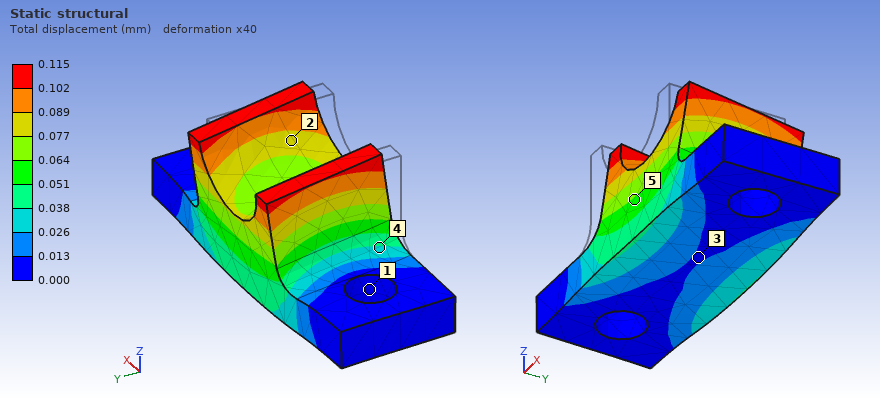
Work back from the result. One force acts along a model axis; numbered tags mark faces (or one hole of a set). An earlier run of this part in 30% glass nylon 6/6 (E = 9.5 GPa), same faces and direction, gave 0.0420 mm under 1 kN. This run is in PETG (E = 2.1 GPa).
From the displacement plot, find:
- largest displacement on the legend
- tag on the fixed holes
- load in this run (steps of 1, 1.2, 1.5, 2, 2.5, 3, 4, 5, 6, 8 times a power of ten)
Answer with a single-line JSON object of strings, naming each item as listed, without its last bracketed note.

{"largest displacement on the legend": "0.115 mm", "tag on the fixed holes": "1", "load in this run": "600 N"}
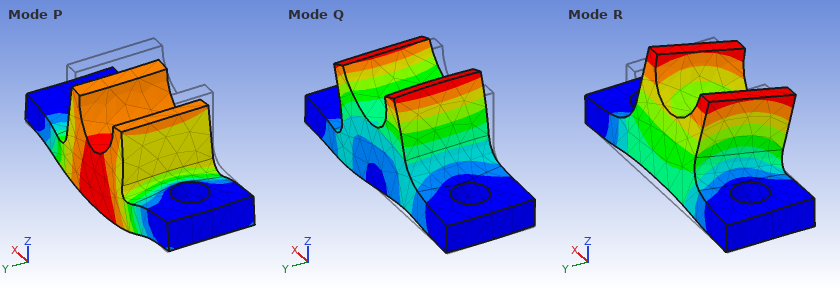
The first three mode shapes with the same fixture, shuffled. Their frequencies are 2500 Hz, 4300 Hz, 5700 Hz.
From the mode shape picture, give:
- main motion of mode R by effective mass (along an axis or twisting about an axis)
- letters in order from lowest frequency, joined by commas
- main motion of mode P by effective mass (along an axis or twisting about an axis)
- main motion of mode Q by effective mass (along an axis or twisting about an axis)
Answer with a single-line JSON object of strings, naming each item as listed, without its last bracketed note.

{"main motion of mode R by effective mass": "along Y", "letters in order from lowest frequency, joined by commas": "R, P, Q", "main motion of mode P by effective mass": "along Z", "main motion of mode Q by effective mass": "along X"}
